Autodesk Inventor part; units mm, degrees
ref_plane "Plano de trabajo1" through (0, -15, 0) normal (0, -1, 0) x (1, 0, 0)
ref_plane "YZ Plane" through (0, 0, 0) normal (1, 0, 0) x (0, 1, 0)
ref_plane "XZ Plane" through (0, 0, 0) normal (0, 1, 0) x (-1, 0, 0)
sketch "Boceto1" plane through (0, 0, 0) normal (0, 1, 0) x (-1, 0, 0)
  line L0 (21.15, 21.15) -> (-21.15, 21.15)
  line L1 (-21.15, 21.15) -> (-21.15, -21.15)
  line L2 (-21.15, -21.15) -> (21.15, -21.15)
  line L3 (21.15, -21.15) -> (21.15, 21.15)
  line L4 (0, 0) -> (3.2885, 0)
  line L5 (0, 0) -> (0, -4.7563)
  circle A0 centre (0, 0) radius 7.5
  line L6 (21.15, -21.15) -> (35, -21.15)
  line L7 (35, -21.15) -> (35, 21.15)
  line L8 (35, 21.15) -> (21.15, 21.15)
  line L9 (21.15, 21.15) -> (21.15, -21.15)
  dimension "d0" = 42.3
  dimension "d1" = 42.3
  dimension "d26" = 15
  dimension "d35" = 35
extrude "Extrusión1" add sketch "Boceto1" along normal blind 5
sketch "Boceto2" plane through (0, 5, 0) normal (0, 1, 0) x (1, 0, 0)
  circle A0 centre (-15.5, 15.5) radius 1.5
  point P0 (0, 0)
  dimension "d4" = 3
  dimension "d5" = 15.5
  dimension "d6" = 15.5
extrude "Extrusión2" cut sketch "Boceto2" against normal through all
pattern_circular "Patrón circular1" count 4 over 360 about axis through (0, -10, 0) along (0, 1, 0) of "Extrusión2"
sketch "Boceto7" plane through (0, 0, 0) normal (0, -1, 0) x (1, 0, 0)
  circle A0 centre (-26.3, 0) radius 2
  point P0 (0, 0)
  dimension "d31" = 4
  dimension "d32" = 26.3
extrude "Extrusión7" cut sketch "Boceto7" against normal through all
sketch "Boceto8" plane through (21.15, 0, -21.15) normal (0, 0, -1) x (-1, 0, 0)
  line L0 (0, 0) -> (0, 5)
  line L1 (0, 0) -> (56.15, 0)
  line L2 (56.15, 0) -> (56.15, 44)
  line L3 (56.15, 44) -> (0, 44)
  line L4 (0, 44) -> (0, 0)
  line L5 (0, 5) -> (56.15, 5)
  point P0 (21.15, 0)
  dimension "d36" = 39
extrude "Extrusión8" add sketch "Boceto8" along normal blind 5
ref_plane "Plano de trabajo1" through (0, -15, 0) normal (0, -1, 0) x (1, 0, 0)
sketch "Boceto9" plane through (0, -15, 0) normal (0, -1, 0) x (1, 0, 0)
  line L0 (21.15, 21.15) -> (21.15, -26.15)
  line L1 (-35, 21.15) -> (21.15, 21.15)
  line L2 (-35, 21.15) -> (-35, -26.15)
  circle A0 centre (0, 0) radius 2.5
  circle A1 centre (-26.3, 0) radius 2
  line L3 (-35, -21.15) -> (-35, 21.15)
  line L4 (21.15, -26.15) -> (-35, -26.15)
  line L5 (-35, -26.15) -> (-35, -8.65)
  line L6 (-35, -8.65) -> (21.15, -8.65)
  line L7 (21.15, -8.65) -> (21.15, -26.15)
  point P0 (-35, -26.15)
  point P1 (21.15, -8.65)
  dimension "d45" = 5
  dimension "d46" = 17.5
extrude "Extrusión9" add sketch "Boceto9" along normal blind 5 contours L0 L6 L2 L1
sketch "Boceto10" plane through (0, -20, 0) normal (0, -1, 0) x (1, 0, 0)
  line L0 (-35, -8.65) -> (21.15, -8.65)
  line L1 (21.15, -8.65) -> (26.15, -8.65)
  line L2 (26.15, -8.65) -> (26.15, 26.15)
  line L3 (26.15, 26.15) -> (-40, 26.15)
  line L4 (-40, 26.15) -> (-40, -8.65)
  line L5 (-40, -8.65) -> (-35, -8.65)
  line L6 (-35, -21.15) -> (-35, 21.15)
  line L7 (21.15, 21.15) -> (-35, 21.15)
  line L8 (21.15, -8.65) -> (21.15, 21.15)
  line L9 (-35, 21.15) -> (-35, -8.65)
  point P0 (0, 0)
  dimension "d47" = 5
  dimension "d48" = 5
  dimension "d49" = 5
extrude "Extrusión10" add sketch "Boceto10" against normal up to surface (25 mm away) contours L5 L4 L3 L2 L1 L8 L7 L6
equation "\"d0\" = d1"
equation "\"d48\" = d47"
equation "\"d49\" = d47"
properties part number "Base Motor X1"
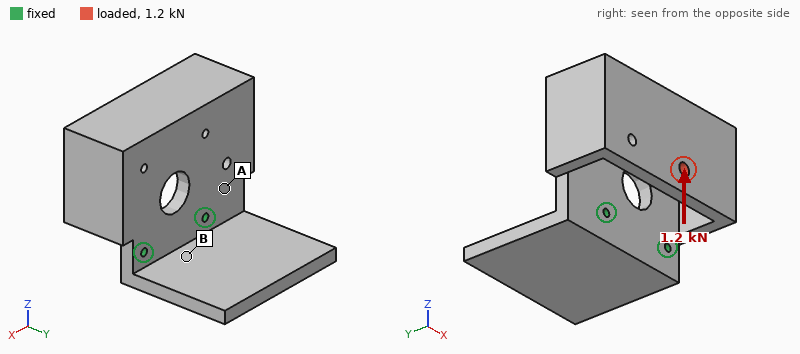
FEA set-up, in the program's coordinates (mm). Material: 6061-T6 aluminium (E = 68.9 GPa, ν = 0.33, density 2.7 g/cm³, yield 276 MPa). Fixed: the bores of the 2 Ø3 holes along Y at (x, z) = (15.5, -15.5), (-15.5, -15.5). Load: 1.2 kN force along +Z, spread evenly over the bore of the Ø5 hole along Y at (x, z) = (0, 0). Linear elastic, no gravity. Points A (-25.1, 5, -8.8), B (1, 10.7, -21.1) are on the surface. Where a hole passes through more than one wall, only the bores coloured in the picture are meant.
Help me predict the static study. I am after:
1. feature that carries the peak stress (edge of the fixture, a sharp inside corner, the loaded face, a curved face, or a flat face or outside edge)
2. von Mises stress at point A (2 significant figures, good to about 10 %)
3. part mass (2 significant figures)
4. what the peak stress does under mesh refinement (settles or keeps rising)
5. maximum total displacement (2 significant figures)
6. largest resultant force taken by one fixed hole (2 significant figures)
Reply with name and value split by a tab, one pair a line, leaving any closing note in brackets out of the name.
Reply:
feature that carries the peak stress	edge of the fixture
von Mises stress at point A	86 MPa
part mass	130 g
what the peak stress does under mesh refinement	keeps rising
maximum total displacement	0.53 mm
largest resultant force taken by one fixed hole	620 N
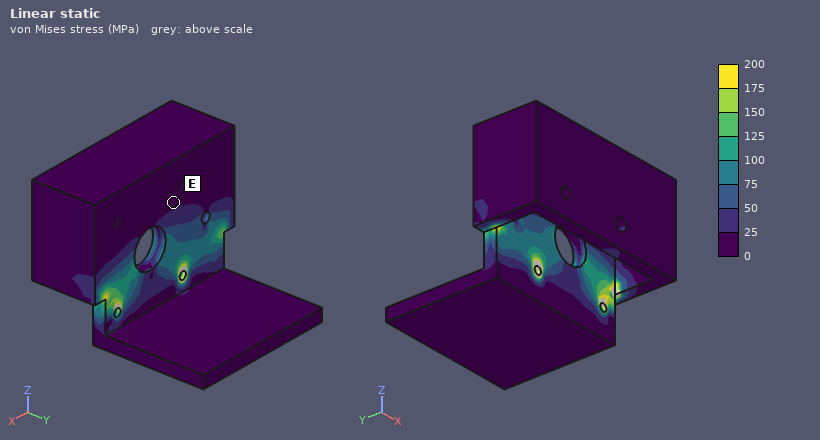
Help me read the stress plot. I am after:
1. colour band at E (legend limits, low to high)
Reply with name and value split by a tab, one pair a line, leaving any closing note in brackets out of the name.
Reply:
colour band at E	0 to 25 MPa
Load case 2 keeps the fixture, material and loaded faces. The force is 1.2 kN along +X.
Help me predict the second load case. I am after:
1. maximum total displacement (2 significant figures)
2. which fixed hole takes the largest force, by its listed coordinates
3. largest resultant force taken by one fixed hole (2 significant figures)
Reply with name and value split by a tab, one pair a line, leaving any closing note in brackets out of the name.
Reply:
maximum total displacement	0.21 mm
which fixed hole takes the largest force, by its listed coordinates	(-15.5, -15.5)
largest resultant force taken by one fixed hole	1.1 kN
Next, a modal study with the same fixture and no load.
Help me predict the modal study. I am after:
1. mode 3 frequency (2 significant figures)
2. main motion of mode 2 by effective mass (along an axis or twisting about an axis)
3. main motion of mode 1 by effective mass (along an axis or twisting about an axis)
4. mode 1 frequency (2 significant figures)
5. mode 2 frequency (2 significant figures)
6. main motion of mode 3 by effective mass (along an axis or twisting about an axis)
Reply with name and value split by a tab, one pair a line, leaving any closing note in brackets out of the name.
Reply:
mode 3 frequency	2000 Hz
main motion of mode 2 by effective mass	along Z
main motion of mode 1 by effective mass	along Y
mode 1 frequency	890 Hz
mode 2 frequency	1700 Hz
main motion of mode 3 by effective mass	along X
